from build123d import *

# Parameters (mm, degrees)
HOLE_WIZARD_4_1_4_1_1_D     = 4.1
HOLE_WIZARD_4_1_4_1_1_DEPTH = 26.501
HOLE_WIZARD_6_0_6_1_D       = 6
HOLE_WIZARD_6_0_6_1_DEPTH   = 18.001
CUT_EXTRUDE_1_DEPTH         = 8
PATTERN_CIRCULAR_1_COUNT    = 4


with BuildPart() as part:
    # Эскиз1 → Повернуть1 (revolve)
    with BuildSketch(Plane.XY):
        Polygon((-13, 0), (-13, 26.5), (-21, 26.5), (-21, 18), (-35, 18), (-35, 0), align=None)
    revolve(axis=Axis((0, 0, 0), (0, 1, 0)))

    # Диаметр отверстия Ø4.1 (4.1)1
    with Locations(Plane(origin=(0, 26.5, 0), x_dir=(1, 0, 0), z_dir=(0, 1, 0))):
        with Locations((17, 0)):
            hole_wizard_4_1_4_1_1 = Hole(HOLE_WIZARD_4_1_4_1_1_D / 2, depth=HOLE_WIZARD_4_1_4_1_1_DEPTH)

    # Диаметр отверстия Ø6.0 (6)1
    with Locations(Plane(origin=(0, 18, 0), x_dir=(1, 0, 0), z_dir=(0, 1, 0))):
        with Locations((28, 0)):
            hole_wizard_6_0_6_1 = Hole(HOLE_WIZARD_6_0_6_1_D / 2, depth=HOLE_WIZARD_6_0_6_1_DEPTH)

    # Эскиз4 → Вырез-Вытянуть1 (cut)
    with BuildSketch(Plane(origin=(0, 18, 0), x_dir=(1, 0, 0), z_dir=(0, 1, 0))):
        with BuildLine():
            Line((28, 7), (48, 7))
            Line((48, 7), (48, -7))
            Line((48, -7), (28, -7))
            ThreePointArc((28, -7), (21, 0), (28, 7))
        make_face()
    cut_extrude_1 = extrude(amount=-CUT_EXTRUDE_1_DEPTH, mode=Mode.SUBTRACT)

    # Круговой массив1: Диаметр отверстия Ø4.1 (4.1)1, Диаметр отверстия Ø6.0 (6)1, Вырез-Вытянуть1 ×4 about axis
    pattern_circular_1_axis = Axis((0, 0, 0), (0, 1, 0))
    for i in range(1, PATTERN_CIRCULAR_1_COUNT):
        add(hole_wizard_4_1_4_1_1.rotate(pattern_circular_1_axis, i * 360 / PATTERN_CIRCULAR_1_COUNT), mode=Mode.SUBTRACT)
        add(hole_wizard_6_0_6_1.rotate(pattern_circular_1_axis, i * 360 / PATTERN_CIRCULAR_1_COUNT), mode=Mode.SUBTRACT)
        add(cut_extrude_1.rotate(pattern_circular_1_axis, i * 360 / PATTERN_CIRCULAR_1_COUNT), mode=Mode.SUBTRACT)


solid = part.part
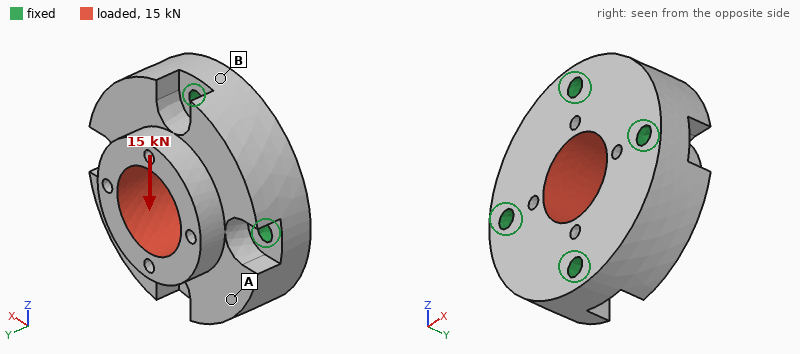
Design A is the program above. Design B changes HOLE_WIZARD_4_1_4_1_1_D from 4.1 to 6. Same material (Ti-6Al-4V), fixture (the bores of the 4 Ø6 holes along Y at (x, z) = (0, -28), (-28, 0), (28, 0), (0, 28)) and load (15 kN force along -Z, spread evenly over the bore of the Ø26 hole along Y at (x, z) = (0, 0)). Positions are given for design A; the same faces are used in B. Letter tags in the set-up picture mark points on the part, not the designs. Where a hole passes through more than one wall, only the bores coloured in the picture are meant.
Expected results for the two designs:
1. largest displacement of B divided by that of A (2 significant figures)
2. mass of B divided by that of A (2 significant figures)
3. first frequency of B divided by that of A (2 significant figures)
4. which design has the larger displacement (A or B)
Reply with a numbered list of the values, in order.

1. 1.3
2. 0.97
3. 0.91
4. B
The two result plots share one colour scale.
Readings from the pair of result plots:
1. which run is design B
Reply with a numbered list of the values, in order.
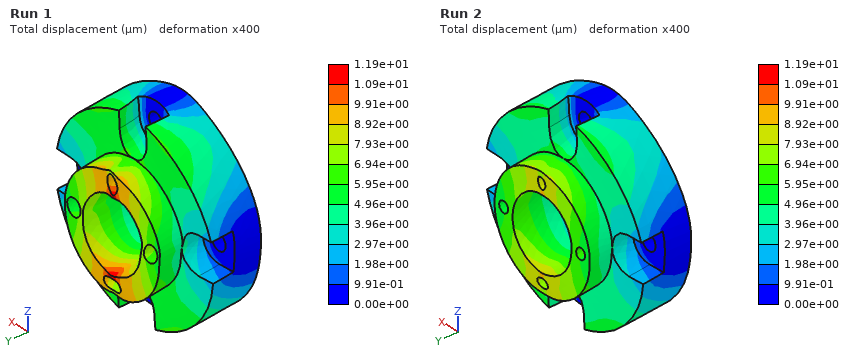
1. Run 1
